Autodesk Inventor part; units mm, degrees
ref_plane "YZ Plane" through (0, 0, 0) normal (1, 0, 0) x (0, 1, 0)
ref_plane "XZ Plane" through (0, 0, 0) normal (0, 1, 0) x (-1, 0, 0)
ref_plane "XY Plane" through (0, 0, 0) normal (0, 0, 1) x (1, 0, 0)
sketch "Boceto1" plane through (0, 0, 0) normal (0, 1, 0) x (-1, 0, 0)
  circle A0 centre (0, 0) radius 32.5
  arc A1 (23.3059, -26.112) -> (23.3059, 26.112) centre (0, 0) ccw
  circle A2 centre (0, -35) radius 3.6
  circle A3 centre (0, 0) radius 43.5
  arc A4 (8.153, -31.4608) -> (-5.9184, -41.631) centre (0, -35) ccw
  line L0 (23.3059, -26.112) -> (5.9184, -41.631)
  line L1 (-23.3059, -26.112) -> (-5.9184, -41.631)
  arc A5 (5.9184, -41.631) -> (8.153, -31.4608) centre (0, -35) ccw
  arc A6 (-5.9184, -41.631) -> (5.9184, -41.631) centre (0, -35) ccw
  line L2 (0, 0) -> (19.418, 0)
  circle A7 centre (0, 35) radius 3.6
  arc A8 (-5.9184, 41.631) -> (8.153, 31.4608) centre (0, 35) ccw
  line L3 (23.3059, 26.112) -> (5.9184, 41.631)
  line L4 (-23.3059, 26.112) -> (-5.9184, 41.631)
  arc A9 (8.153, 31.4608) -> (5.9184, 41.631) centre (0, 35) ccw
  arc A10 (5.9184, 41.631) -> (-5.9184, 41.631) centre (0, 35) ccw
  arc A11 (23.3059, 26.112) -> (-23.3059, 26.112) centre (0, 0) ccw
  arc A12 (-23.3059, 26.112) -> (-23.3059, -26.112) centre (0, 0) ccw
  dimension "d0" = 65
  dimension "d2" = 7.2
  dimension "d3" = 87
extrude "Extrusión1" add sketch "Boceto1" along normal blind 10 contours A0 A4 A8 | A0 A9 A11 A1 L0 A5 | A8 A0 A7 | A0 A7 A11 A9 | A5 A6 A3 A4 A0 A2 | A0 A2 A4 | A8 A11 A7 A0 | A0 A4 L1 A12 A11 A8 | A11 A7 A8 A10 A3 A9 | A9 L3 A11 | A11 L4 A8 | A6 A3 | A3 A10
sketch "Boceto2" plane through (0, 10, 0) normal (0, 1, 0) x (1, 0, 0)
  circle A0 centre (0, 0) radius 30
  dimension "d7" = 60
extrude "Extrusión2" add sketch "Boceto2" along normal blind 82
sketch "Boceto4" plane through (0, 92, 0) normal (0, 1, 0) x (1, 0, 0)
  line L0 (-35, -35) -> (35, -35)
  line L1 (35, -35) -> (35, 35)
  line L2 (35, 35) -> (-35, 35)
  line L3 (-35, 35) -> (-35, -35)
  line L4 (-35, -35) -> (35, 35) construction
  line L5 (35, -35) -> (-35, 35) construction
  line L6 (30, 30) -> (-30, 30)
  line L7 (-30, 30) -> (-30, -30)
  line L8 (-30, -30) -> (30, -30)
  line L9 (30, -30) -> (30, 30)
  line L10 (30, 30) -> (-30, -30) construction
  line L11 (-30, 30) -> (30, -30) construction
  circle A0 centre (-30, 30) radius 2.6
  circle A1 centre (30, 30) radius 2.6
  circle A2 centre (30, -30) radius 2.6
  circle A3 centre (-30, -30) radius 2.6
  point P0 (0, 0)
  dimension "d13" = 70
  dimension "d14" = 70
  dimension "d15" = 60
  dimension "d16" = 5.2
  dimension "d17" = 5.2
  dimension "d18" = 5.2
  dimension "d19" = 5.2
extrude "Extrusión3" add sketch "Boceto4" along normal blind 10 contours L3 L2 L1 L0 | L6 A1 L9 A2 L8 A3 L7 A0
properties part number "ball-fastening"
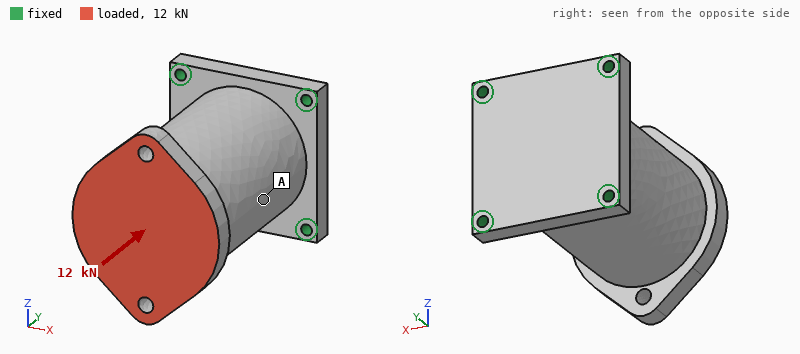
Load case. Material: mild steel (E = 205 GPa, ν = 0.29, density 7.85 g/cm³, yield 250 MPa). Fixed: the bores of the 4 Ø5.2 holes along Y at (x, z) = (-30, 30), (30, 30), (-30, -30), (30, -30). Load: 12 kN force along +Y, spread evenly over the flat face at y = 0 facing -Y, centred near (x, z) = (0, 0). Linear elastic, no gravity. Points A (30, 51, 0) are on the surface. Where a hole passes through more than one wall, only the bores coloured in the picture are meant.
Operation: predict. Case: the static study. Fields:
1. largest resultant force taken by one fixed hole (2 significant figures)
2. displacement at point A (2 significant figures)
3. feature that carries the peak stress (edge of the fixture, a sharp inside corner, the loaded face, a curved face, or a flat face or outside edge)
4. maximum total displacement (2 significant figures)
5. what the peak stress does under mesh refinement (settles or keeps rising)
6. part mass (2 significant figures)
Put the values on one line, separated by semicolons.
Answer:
3.1 kN; 7.7 µm; edge of the fixture; 11 µm; keeps rising; 2.5 kg
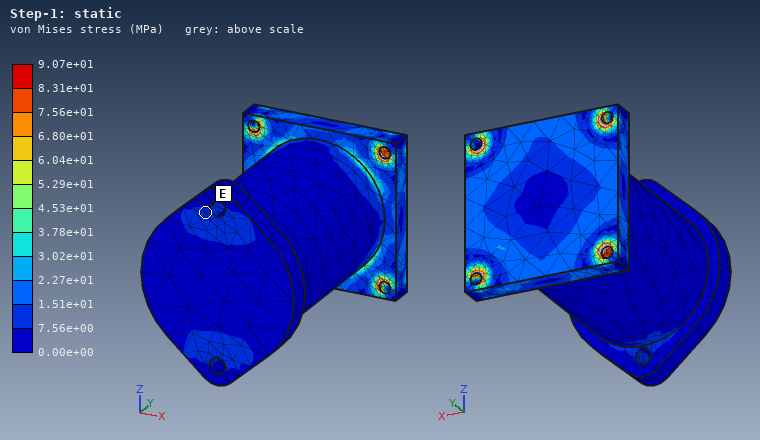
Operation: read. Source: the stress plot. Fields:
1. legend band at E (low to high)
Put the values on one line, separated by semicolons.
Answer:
7.56e+00 to 1.51e+01 MPa
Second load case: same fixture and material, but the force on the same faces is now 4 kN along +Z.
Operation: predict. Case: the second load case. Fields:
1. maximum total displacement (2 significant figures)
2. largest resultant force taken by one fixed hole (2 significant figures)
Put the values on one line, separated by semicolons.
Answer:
46 µm; 3.8 kN
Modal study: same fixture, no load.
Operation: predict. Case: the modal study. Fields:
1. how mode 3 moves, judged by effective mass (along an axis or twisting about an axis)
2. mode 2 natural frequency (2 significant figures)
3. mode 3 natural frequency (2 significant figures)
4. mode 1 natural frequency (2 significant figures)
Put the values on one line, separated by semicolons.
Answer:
along Y; 1700 Hz; 4100 Hz; 1700 Hz
